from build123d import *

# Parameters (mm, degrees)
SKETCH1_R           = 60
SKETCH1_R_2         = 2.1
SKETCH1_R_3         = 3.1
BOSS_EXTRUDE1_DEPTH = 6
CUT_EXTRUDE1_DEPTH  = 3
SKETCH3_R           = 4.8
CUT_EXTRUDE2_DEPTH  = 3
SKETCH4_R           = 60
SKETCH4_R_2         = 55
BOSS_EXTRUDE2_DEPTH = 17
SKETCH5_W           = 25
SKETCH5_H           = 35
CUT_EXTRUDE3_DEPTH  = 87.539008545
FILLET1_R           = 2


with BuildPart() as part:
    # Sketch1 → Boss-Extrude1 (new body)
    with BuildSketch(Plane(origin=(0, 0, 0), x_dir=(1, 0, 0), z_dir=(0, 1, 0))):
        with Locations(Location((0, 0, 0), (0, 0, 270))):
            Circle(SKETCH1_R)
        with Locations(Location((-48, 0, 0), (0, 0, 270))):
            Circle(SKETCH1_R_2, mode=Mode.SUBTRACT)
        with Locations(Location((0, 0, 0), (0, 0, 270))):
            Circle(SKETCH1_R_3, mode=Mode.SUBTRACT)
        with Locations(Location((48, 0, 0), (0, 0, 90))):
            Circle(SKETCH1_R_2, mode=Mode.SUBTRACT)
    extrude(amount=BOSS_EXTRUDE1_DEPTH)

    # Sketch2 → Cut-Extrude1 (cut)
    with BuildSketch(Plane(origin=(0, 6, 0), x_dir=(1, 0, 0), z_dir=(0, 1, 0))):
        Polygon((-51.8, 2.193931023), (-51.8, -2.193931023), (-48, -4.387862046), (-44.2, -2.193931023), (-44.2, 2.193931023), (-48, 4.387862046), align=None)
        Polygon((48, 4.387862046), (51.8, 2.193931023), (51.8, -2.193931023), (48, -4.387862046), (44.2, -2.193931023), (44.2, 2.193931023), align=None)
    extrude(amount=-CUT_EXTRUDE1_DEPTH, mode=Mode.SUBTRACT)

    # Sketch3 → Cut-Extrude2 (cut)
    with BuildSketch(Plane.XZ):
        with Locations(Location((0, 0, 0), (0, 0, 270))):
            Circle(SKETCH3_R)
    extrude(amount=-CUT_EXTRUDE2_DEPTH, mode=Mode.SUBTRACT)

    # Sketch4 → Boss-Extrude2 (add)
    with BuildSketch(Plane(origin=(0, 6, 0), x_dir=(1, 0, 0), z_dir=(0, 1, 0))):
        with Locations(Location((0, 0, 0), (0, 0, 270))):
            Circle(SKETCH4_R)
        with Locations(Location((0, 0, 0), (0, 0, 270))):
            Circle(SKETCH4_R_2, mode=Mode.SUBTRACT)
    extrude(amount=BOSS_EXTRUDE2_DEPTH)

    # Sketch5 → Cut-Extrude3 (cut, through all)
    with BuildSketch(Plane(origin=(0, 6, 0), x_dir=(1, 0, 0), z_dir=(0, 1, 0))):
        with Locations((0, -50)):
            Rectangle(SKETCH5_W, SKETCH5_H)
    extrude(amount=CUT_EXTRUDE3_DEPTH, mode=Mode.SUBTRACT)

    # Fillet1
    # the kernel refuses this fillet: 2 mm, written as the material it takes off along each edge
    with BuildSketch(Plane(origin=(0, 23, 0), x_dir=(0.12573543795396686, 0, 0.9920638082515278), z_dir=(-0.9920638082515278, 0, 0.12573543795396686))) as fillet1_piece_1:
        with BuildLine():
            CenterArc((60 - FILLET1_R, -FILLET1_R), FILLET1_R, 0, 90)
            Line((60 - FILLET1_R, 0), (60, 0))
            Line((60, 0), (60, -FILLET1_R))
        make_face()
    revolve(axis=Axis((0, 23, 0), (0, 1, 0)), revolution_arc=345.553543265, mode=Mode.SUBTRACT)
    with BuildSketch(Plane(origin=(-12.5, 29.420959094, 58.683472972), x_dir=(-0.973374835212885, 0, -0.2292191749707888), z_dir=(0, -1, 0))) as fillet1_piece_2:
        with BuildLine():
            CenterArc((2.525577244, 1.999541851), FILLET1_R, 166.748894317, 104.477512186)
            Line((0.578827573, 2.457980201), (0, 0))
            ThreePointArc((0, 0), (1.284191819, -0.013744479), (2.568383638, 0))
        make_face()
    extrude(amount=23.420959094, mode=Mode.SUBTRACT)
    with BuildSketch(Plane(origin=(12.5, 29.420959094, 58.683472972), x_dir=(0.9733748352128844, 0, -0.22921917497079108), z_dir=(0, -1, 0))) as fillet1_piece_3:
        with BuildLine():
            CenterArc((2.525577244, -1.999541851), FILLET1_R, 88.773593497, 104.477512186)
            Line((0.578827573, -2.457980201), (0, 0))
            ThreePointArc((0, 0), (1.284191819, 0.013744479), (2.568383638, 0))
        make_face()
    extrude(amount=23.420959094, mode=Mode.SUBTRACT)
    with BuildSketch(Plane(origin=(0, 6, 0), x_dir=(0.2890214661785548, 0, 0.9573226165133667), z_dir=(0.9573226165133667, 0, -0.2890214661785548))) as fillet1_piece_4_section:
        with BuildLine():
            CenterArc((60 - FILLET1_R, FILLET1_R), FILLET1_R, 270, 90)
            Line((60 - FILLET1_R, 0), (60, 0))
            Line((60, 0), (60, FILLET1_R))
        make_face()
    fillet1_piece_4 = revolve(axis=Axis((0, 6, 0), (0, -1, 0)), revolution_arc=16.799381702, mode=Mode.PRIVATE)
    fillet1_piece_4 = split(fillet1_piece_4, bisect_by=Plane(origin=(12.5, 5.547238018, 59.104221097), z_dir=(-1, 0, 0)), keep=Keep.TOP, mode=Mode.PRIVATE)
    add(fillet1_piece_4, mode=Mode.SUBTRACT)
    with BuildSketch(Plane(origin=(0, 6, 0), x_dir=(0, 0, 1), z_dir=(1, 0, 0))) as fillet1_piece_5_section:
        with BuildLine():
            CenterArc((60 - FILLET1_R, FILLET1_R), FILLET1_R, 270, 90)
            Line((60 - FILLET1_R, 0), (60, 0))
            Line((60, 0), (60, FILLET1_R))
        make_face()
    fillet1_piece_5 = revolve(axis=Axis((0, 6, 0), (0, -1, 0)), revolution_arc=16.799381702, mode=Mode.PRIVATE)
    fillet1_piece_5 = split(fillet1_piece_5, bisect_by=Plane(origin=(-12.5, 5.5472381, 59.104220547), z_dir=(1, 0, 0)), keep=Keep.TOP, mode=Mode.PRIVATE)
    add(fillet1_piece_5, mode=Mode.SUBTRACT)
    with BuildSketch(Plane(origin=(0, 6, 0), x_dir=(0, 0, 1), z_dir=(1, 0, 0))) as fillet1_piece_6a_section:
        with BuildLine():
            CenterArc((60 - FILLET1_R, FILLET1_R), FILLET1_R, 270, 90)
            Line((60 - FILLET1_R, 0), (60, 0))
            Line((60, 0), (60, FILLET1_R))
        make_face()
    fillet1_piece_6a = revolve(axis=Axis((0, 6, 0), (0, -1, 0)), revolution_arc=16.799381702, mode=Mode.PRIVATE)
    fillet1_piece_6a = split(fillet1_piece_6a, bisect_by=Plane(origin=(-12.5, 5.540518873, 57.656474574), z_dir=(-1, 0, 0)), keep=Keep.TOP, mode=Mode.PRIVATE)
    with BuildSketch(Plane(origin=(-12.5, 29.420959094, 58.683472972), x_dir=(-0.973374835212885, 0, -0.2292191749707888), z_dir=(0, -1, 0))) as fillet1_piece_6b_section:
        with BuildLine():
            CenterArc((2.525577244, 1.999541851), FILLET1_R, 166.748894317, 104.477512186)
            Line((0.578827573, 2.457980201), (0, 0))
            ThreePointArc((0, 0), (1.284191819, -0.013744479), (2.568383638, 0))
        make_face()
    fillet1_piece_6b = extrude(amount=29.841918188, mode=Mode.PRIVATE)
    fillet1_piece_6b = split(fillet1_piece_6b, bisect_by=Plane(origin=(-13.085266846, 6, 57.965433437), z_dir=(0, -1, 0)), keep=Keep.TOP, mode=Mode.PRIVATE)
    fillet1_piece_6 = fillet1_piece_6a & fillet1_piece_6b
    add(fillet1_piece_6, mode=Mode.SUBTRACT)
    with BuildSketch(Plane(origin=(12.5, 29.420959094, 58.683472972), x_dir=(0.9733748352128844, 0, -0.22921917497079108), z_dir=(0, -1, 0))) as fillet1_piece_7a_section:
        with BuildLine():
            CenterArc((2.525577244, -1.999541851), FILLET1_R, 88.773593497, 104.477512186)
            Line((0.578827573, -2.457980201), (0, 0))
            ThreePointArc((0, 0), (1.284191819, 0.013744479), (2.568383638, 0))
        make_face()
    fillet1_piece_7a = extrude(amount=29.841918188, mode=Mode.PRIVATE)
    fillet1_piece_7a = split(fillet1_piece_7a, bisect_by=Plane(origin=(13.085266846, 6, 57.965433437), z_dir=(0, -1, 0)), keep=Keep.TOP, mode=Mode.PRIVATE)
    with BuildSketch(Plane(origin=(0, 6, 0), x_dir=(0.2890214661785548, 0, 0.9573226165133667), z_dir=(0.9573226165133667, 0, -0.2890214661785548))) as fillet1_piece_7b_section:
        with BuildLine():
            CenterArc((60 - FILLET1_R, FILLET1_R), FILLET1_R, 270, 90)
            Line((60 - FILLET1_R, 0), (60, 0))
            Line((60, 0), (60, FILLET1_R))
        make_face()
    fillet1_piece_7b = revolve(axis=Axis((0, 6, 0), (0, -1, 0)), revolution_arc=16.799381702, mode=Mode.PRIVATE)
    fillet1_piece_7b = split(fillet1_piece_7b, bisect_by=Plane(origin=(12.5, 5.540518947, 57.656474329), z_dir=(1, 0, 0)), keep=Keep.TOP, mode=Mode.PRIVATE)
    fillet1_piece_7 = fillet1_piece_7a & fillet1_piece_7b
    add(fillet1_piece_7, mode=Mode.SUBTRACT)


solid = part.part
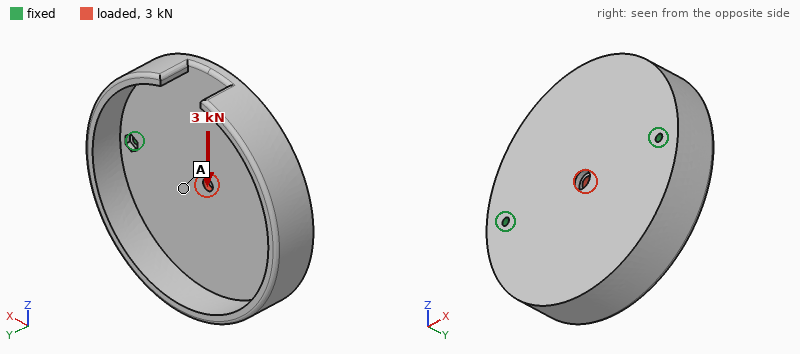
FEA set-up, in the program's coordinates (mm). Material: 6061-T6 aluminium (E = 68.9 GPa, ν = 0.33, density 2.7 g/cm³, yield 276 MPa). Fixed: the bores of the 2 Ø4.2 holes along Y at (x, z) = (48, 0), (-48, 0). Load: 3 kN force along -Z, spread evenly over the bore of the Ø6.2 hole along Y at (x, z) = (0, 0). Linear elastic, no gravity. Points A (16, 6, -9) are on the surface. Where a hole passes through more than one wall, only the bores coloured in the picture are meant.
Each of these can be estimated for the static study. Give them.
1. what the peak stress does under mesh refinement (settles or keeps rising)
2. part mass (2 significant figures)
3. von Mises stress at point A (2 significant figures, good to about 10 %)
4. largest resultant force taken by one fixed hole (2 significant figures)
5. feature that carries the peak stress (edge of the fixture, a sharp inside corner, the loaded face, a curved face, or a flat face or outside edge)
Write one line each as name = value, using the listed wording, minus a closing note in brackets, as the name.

what the peak stress does under mesh refinement = keeps rising
part mass = 260 g
von Mises stress at point A = 8.1 MPa
largest resultant force taken by one fixed hole = 1.5 kN
feature that carries the peak stress = edge of the fixture
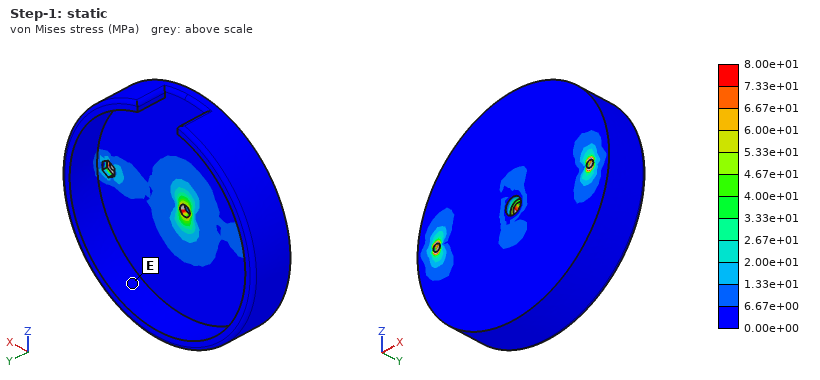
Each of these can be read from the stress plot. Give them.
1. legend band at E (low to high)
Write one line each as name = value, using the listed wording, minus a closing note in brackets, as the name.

legend band at E = 0.00e+00 to 6.67e+00 MPa
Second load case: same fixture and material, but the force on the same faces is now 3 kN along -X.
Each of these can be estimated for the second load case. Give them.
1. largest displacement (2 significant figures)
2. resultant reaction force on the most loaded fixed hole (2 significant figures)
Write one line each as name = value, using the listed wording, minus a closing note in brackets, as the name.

largest displacement = 12 µm
resultant reaction force on the most loaded fixed hole = 1.5 kN
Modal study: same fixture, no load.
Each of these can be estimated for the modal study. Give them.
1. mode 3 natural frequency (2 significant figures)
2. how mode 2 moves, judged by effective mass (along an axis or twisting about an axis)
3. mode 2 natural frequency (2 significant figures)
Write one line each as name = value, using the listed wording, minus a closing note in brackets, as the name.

mode 3 natural frequency = 2500 Hz
how mode 2 moves, judged by effective mass = along Y
mode 2 natural frequency = 1600 Hz
